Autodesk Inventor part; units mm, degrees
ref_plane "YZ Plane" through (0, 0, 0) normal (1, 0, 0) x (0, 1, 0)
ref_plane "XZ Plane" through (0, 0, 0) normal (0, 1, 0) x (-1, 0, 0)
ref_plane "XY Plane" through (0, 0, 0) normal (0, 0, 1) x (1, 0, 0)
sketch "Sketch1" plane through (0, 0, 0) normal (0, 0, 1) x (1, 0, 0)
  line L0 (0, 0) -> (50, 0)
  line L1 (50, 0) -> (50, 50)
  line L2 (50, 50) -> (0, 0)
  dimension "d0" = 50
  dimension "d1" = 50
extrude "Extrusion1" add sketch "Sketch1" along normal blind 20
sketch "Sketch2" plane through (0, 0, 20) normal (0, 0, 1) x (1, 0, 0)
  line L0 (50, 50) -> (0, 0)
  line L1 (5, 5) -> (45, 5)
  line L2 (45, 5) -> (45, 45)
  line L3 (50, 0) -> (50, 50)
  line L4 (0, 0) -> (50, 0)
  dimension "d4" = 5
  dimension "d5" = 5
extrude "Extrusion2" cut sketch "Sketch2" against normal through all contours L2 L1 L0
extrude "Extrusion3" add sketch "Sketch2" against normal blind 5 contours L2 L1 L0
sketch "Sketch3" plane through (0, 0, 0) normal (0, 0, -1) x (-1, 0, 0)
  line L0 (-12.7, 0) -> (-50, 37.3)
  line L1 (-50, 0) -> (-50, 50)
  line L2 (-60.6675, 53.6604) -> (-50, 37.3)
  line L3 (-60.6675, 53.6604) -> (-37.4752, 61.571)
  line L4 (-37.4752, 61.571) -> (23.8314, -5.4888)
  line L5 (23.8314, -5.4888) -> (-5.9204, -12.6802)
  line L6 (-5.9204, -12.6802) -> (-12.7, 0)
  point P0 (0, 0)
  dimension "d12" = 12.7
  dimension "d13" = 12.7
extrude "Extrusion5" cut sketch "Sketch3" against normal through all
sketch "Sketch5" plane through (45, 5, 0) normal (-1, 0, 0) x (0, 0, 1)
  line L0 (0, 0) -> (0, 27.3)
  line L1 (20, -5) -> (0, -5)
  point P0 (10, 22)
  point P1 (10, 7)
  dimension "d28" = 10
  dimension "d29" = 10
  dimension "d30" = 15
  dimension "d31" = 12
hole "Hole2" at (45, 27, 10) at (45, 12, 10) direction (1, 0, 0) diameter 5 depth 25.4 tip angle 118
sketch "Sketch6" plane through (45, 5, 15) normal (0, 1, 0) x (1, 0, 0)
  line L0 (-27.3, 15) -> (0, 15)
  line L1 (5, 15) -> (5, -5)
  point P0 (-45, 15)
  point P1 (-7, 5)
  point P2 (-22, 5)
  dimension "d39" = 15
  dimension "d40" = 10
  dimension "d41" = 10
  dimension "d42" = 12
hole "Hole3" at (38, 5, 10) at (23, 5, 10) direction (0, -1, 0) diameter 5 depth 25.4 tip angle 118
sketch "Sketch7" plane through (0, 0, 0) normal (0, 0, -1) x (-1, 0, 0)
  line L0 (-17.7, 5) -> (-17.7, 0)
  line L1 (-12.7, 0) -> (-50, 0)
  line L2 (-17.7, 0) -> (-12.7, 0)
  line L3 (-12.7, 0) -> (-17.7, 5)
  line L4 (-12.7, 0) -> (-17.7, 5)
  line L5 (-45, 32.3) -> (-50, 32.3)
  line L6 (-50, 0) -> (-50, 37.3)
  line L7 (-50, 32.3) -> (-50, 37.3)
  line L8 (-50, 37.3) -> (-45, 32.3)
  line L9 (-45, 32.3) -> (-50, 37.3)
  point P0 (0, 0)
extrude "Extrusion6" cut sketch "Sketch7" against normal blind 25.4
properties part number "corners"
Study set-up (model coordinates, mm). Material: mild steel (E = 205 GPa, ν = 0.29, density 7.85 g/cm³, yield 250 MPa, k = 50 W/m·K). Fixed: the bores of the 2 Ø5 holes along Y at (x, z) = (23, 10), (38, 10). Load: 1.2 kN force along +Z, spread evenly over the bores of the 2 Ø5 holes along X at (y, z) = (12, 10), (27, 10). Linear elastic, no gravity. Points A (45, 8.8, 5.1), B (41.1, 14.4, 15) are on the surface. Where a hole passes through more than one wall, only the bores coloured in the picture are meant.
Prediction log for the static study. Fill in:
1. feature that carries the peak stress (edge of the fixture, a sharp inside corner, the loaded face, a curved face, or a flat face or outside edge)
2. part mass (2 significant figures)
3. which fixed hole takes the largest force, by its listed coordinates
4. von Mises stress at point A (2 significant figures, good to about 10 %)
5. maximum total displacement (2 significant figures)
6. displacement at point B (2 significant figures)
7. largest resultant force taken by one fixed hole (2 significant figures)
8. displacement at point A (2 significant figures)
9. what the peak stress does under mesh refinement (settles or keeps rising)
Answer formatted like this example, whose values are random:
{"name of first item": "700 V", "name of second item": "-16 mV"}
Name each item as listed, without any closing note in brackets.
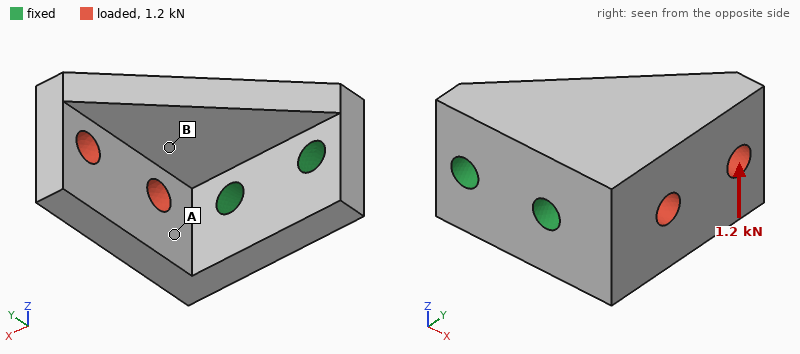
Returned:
{"feature that carries the peak stress": "edge of the fixture", "part mass": "58 g", "which fixed hole takes the largest force, by its listed coordinates": "(38, 10)", "von Mises stress at point A": "64 MPa", "maximum total displacement": "58 µm", "displacement at point B": "20 µm", "largest resultant force taken by one fixed hole": "1.6 kN", "displacement at point A": "15 µm", "what the peak stress does under mesh refinement": "keeps rising"}
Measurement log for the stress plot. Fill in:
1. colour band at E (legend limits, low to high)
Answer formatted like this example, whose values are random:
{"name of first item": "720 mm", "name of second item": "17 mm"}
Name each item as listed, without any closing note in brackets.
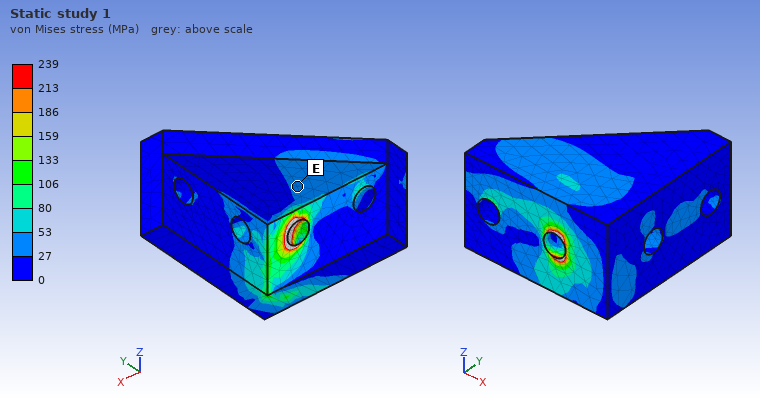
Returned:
{"colour band at E": "27 to 53 MPa"}
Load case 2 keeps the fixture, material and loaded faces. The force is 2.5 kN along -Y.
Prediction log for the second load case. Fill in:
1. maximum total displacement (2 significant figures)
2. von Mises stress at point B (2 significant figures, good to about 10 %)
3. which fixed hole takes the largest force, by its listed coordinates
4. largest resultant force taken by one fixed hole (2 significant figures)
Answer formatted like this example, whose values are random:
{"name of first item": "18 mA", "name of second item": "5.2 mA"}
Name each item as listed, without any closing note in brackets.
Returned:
{"maximum total displacement": "26 µm", "von Mises stress at point B": "24 MPa", "which fixed hole takes the largest force, by its listed coordinates": "(38, 10)", "largest resultant force taken by one fixed hole": "3.2 kN"}
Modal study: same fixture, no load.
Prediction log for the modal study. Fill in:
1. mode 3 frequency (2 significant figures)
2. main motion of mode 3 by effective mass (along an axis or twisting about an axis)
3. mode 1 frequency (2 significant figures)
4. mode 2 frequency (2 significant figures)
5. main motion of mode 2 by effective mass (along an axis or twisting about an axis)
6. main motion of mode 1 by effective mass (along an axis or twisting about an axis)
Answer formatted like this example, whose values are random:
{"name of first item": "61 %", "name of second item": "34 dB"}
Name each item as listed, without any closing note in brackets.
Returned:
{"mode 3 frequency": "15 kHz", "main motion of mode 3 by effective mass": "along Y", "mode 1 frequency": "5300 Hz", "mode 2 frequency": "7700 Hz", "main motion of mode 2 by effective mass": "along X", "main motion of mode 1 by effective mass": "along Z"}
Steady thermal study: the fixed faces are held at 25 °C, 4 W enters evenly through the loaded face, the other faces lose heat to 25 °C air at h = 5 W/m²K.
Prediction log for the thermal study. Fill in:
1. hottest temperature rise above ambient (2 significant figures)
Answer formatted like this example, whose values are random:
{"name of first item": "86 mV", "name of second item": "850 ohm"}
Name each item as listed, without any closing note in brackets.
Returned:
{"hottest temperature rise above ambient": "14 K"}
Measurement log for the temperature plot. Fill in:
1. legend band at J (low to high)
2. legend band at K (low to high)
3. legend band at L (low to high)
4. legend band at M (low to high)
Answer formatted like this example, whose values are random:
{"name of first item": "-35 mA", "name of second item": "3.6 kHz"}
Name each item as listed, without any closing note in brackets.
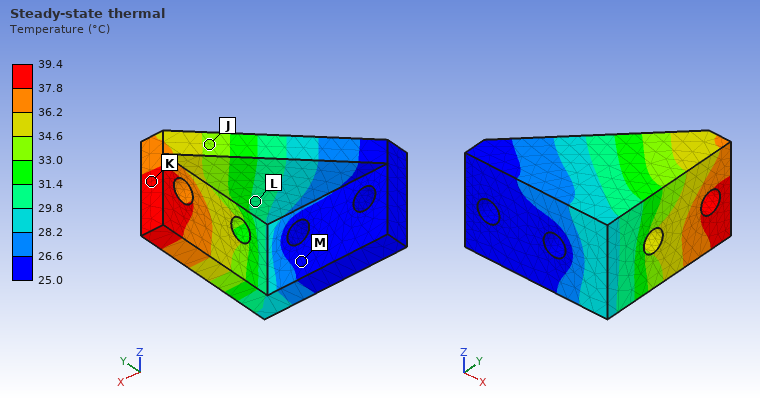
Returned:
{"legend band at J": "33.0 to 34.6 °C", "legend band at K": "37.8 to 39.4 °C", "legend band at L": "29.8 to 31.4 °C", "legend band at M": "25.0 to 26.6 °C"}
